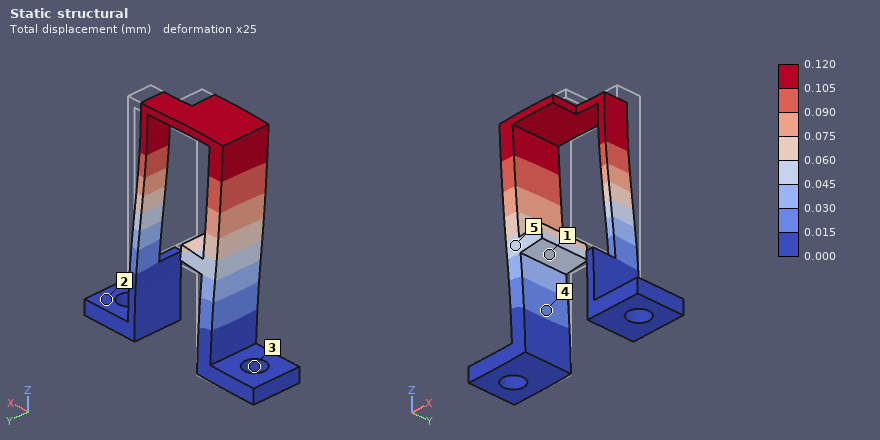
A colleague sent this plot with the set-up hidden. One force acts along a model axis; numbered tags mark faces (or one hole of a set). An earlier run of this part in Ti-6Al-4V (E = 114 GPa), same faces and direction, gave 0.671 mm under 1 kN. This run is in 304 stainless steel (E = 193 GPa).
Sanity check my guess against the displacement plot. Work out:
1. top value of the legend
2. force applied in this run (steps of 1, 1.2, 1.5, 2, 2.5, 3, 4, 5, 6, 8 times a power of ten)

0.120 mm
300 N
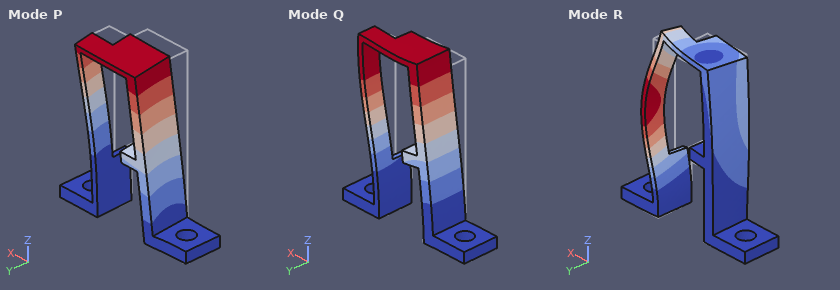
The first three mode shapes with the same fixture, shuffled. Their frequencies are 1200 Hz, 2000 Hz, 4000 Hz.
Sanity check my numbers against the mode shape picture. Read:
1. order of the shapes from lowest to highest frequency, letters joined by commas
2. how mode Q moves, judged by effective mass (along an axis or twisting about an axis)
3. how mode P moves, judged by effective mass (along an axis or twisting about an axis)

Q, P, R
along X
along Y
